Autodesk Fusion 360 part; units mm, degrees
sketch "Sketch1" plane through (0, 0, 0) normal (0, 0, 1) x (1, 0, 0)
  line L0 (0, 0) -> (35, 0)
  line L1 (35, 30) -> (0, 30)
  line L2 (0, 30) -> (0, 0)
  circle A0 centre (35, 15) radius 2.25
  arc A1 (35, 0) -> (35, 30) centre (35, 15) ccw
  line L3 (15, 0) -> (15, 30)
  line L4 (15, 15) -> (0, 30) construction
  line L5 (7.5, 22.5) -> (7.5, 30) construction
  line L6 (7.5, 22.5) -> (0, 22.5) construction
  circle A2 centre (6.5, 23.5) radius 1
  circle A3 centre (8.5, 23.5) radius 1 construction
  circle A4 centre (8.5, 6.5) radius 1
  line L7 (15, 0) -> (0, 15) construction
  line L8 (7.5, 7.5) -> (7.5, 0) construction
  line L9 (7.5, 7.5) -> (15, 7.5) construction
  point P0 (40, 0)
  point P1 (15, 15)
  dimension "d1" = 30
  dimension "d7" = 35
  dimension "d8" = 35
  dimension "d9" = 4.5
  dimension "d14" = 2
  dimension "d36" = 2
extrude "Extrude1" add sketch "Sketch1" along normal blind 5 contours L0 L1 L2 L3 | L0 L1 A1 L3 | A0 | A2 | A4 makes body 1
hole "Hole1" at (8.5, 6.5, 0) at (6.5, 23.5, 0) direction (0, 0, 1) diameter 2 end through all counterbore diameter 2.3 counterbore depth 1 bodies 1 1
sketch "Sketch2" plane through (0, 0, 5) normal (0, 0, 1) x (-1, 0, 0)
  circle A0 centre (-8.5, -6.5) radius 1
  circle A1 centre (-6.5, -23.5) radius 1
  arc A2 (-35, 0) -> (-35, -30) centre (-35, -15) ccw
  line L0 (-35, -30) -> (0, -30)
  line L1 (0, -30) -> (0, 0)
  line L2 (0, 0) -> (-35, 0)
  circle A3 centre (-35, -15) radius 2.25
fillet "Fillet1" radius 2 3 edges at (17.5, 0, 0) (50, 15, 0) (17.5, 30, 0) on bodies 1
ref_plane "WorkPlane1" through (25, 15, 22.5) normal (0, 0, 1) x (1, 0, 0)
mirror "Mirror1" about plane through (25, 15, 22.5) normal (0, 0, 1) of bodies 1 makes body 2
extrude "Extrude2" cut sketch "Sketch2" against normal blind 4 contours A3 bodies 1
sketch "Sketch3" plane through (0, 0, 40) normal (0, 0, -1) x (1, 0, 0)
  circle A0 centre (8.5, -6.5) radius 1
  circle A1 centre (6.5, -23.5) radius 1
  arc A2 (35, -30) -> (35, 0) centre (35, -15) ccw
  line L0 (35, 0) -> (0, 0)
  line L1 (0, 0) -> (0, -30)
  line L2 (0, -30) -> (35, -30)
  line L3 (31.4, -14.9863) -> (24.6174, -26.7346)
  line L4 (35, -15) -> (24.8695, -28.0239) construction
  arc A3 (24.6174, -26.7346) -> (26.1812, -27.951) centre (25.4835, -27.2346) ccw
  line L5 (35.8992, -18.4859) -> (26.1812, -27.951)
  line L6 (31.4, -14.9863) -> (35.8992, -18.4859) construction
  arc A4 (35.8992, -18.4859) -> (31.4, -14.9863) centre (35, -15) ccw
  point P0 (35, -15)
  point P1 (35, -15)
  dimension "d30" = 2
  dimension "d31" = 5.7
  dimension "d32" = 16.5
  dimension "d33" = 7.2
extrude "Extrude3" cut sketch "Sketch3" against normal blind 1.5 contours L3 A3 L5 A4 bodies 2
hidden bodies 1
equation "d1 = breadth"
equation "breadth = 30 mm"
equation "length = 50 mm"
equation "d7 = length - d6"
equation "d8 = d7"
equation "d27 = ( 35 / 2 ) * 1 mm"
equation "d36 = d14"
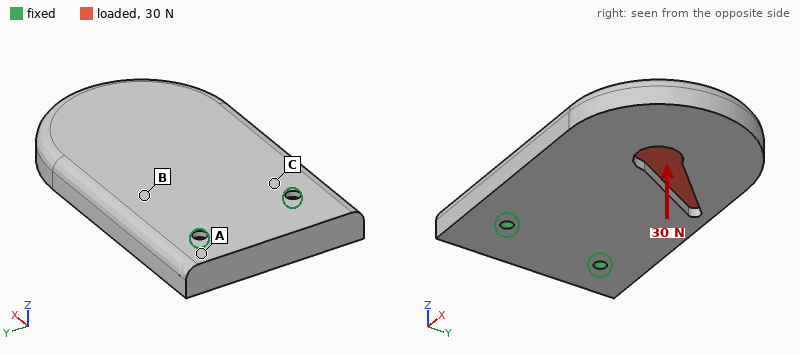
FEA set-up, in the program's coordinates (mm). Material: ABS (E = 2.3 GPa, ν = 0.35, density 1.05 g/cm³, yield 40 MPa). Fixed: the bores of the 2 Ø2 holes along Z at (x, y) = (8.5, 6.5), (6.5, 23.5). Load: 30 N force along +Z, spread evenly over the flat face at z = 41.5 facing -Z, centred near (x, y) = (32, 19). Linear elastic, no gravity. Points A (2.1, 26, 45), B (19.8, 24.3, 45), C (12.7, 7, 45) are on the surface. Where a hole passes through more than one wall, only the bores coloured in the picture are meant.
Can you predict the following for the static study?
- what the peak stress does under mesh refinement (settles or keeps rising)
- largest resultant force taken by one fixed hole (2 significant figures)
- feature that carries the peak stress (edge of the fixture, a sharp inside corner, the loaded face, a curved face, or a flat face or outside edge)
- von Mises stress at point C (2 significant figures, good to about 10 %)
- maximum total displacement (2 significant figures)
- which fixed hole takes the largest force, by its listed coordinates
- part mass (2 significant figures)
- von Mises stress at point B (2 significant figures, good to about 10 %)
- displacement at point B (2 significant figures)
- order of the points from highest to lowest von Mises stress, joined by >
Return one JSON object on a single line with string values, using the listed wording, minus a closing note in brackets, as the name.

{"what the peak stress does under mesh refinement": "keeps rising", "largest resultant force taken by one fixed hole": "16 N", "feature that carries the peak stress": "edge of the fixture", "von Mises stress at point C": "5.2 MPa", "maximum total displacement": "0.63 mm", "which fixed hole takes the largest force, by its listed coordinates": "(6.5, 23.5)", "part mass": "7.1 g", "von Mises stress at point B": "2.9 MPa", "displacement at point B": "0.14 mm", "order of the points from highest to lowest von Mises stress, joined by >": "C > B > A"}
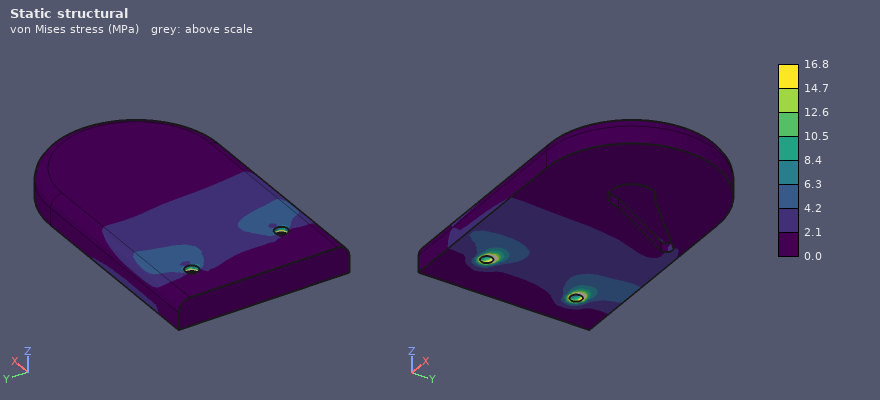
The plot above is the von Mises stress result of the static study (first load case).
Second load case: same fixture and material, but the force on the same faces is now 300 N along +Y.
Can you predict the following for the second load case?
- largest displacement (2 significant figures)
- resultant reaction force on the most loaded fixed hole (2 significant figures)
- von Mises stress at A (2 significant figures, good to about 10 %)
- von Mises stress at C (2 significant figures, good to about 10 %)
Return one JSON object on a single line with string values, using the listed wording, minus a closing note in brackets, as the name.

{"largest displacement": "0.31 mm", "resultant reaction force on the most loaded fixed hole": "450 N", "von Mises stress at A": "4.4 MPa", "von Mises stress at C": "7.4 MPa"}
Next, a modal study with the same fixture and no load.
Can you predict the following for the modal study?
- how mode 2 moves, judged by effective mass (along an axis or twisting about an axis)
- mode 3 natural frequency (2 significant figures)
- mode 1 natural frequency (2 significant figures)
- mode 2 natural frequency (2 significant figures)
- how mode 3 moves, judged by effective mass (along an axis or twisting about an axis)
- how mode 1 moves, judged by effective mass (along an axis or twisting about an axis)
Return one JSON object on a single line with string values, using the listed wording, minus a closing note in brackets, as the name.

{"how mode 2 moves, judged by effective mass": "twisting about X", "mode 3 natural frequency": "2800 Hz", "mode 1 natural frequency": "660 Hz", "mode 2 natural frequency": "2200 Hz", "how mode 3 moves, judged by effective mass": "along Y", "how mode 1 moves, judged by effective mass": "along Z"}
